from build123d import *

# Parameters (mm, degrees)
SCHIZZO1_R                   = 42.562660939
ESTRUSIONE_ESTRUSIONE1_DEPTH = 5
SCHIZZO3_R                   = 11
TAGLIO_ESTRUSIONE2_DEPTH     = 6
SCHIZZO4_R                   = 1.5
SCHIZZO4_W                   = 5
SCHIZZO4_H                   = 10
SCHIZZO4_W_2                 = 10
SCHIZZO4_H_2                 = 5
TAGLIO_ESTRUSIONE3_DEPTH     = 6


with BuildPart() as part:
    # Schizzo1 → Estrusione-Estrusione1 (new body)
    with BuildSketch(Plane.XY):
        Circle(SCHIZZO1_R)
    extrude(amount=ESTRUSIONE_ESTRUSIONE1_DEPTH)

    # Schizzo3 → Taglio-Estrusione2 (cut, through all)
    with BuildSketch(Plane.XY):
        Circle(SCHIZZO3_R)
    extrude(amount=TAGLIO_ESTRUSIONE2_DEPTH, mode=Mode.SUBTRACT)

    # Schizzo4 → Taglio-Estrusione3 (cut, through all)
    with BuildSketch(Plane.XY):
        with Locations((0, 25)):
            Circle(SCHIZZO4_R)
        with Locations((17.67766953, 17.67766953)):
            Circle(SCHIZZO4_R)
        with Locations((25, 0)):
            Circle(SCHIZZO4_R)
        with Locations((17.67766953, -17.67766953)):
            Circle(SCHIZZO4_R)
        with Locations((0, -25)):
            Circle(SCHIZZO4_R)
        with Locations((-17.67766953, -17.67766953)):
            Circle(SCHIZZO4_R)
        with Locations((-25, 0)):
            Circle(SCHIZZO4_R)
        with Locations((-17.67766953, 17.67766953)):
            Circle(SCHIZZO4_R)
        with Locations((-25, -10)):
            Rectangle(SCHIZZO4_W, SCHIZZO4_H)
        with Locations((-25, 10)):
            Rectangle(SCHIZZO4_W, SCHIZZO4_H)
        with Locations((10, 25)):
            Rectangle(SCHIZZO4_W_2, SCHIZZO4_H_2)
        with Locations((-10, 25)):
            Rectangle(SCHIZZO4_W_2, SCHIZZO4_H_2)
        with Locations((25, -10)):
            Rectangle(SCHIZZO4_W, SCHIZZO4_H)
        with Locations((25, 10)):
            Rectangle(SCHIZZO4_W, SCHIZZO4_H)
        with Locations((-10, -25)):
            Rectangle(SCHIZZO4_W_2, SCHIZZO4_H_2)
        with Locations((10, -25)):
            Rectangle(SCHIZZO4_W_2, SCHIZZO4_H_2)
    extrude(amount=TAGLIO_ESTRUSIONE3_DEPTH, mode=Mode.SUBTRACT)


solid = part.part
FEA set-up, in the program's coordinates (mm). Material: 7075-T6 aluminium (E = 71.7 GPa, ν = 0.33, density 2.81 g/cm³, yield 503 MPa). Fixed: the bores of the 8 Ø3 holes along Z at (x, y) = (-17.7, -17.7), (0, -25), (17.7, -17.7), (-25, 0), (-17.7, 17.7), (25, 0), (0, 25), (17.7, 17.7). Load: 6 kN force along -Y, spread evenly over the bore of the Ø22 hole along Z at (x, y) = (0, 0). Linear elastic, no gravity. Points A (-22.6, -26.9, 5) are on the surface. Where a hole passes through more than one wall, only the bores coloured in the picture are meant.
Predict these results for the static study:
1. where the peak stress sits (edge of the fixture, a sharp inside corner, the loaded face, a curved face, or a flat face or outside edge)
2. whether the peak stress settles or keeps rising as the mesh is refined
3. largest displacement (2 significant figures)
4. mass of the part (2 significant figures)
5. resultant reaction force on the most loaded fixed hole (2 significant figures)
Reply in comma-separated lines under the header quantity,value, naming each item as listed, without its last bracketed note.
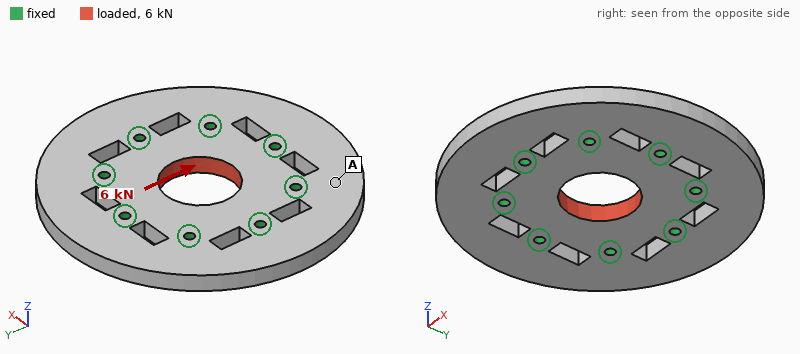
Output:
quantity,value
where the peak stress sits,edge of the fixture
whether the peak stress settles or keeps rising as the mesh is refined,keeps rising
largest displacement,4.4 µm
mass of the part,68 g
resultant reaction force on the most loaded fixed hole,1.2 kN
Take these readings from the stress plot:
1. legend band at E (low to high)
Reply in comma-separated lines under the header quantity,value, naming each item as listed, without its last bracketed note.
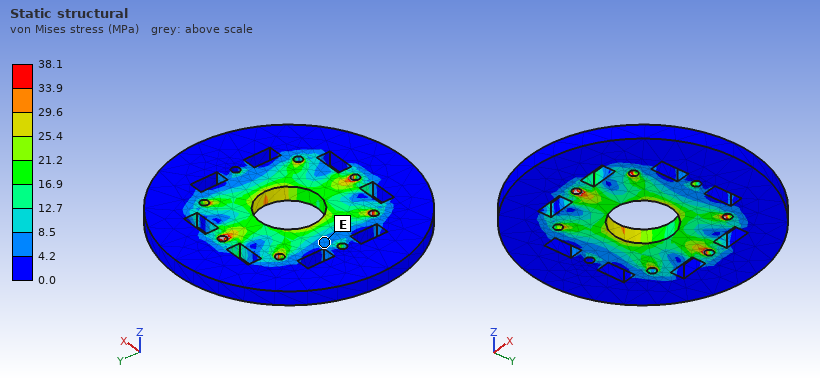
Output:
quantity,value
legend band at E,4.2 to 8.5 MPa
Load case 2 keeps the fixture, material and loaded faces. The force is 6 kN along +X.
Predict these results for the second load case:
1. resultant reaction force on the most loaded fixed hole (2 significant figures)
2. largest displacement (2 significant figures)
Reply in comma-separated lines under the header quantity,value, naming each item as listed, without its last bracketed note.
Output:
quantity,value
resultant reaction force on the most loaded fixed hole,1.2 kN
largest displacement,4.4 µm
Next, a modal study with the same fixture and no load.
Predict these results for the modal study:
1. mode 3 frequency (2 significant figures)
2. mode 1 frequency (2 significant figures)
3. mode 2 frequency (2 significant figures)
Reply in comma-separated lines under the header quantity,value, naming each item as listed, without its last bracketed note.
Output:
quantity,value
mode 3 frequency,9400 Hz
mode 1 frequency,9200 Hz
mode 2 frequency,9400 Hz
